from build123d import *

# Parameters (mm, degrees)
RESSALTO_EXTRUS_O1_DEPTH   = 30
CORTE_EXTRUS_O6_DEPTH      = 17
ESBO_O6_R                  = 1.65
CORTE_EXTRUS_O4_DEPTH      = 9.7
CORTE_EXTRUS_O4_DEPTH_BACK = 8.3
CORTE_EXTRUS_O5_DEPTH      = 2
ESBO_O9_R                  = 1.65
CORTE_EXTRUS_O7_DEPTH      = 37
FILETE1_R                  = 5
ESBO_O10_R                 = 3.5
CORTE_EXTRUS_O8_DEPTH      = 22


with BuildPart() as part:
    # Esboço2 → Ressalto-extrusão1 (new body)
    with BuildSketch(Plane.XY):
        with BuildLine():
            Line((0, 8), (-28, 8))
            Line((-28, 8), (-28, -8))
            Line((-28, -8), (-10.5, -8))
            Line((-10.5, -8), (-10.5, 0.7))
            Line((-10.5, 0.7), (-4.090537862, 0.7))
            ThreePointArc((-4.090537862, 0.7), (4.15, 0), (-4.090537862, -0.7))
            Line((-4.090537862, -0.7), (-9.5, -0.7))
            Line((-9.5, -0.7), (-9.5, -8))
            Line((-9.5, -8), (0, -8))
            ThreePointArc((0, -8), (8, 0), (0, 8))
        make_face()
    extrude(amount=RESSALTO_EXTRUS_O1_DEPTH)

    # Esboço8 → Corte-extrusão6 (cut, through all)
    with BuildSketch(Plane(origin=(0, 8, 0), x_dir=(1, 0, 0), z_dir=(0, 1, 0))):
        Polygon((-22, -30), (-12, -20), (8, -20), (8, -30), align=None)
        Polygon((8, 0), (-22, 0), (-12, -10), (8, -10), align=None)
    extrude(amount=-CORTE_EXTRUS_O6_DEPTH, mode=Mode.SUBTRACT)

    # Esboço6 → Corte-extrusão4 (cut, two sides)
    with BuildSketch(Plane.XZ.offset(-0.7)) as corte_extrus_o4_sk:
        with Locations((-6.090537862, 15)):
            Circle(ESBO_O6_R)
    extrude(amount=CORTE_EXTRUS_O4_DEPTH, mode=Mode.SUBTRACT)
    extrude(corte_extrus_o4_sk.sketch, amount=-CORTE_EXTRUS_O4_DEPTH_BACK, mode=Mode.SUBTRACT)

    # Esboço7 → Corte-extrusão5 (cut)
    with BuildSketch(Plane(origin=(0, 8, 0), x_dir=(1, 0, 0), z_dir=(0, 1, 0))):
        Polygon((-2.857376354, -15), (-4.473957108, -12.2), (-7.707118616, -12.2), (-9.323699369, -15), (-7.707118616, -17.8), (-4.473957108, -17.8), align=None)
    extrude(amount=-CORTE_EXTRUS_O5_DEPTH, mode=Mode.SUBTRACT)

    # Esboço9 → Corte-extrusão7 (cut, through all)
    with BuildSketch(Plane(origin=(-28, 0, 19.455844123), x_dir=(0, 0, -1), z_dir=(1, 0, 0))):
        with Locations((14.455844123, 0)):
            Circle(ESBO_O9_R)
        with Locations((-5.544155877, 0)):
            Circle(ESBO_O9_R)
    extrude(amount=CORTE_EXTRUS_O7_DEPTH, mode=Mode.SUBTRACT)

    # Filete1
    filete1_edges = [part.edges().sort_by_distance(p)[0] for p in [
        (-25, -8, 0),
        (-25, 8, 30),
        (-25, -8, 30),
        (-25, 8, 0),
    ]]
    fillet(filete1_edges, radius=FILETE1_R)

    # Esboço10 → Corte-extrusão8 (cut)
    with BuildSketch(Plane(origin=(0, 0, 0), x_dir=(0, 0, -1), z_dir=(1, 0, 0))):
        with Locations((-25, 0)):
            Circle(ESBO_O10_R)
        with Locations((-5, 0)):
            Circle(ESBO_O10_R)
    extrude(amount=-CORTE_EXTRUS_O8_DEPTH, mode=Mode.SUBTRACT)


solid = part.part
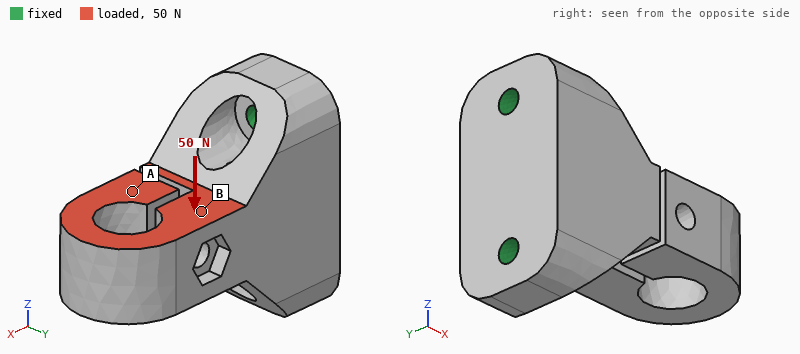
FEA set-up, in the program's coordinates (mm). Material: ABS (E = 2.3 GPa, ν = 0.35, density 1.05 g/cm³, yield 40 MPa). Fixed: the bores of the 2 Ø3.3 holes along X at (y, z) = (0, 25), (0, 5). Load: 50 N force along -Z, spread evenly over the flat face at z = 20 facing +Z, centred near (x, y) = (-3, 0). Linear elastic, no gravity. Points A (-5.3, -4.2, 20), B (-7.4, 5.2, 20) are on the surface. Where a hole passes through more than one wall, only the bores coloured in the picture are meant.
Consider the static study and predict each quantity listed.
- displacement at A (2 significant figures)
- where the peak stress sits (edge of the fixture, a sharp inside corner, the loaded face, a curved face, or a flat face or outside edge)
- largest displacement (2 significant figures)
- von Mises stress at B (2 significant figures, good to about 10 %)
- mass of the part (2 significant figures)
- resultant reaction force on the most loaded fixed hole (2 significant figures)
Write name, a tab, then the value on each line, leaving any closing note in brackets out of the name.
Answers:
displacement at A	0.40 mm
where the peak stress sits	a curved face
largest displacement	0.51 mm
von Mises stress at B	4.2 MPa
mass of the part	7.9 g
resultant reaction force on the most loaded fixed hole	58 N
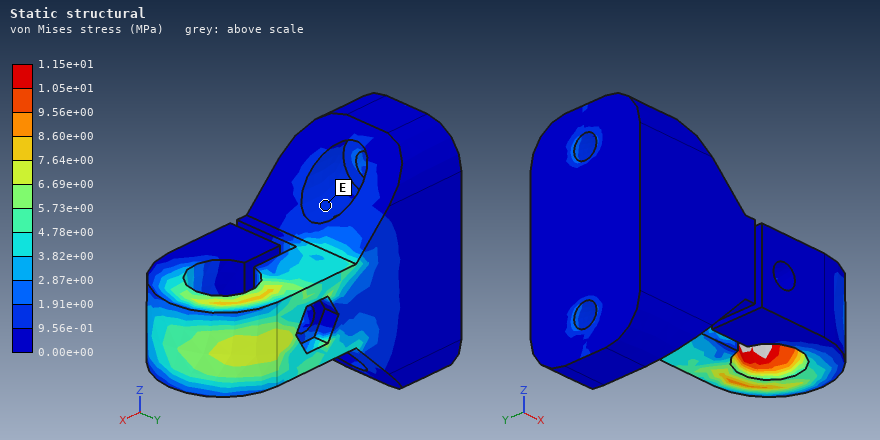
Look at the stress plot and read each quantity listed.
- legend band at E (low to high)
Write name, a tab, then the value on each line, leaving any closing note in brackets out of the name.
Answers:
legend band at E	9.56e-01 to 1.91e+00 MPa
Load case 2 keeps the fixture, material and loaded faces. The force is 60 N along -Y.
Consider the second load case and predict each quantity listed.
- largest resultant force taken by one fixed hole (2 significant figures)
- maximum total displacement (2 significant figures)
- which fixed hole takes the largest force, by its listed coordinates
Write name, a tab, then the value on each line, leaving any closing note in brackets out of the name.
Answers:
largest resultant force taken by one fixed hole	44 N
maximum total displacement	0.58 mm
which fixed hole takes the largest force, by its listed coordinates	(0, 25)
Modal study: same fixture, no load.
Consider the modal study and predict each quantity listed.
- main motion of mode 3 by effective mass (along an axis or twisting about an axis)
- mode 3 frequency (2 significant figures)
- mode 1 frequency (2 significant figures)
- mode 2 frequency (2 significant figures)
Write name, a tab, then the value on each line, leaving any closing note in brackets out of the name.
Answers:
main motion of mode 3 by effective mass	along Y
mode 3 frequency	1600 Hz
mode 1 frequency	1200 Hz
mode 2 frequency	1300 Hz
